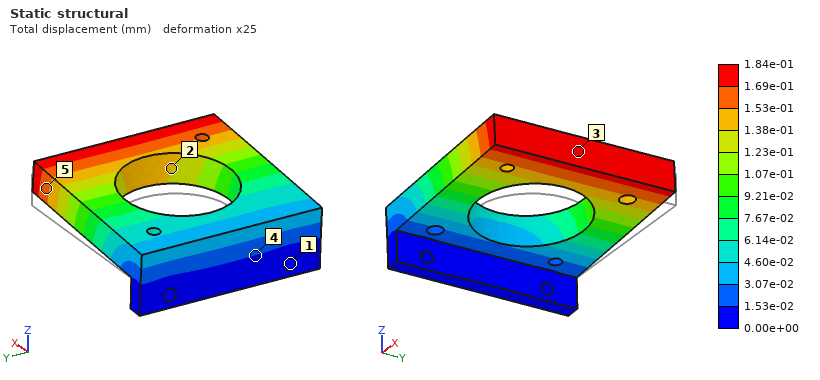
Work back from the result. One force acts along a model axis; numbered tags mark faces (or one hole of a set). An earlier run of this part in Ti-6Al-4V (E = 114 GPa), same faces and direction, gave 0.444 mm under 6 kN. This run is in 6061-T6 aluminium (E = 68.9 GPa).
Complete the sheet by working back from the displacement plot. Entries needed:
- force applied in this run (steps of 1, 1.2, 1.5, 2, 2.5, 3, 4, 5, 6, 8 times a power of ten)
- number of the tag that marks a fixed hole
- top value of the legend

1.5 kN
1
1.84e-01 mm
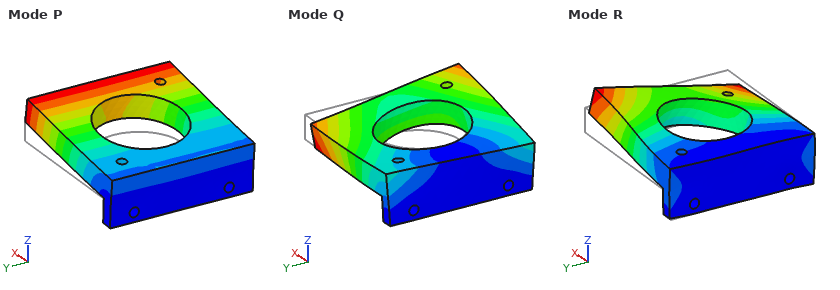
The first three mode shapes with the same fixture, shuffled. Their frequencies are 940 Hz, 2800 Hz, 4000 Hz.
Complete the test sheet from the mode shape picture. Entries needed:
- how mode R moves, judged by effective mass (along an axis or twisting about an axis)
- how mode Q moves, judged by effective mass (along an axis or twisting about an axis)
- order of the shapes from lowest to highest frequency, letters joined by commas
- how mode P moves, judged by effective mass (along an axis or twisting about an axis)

along Y
along Y
P, Q, R
along Z
